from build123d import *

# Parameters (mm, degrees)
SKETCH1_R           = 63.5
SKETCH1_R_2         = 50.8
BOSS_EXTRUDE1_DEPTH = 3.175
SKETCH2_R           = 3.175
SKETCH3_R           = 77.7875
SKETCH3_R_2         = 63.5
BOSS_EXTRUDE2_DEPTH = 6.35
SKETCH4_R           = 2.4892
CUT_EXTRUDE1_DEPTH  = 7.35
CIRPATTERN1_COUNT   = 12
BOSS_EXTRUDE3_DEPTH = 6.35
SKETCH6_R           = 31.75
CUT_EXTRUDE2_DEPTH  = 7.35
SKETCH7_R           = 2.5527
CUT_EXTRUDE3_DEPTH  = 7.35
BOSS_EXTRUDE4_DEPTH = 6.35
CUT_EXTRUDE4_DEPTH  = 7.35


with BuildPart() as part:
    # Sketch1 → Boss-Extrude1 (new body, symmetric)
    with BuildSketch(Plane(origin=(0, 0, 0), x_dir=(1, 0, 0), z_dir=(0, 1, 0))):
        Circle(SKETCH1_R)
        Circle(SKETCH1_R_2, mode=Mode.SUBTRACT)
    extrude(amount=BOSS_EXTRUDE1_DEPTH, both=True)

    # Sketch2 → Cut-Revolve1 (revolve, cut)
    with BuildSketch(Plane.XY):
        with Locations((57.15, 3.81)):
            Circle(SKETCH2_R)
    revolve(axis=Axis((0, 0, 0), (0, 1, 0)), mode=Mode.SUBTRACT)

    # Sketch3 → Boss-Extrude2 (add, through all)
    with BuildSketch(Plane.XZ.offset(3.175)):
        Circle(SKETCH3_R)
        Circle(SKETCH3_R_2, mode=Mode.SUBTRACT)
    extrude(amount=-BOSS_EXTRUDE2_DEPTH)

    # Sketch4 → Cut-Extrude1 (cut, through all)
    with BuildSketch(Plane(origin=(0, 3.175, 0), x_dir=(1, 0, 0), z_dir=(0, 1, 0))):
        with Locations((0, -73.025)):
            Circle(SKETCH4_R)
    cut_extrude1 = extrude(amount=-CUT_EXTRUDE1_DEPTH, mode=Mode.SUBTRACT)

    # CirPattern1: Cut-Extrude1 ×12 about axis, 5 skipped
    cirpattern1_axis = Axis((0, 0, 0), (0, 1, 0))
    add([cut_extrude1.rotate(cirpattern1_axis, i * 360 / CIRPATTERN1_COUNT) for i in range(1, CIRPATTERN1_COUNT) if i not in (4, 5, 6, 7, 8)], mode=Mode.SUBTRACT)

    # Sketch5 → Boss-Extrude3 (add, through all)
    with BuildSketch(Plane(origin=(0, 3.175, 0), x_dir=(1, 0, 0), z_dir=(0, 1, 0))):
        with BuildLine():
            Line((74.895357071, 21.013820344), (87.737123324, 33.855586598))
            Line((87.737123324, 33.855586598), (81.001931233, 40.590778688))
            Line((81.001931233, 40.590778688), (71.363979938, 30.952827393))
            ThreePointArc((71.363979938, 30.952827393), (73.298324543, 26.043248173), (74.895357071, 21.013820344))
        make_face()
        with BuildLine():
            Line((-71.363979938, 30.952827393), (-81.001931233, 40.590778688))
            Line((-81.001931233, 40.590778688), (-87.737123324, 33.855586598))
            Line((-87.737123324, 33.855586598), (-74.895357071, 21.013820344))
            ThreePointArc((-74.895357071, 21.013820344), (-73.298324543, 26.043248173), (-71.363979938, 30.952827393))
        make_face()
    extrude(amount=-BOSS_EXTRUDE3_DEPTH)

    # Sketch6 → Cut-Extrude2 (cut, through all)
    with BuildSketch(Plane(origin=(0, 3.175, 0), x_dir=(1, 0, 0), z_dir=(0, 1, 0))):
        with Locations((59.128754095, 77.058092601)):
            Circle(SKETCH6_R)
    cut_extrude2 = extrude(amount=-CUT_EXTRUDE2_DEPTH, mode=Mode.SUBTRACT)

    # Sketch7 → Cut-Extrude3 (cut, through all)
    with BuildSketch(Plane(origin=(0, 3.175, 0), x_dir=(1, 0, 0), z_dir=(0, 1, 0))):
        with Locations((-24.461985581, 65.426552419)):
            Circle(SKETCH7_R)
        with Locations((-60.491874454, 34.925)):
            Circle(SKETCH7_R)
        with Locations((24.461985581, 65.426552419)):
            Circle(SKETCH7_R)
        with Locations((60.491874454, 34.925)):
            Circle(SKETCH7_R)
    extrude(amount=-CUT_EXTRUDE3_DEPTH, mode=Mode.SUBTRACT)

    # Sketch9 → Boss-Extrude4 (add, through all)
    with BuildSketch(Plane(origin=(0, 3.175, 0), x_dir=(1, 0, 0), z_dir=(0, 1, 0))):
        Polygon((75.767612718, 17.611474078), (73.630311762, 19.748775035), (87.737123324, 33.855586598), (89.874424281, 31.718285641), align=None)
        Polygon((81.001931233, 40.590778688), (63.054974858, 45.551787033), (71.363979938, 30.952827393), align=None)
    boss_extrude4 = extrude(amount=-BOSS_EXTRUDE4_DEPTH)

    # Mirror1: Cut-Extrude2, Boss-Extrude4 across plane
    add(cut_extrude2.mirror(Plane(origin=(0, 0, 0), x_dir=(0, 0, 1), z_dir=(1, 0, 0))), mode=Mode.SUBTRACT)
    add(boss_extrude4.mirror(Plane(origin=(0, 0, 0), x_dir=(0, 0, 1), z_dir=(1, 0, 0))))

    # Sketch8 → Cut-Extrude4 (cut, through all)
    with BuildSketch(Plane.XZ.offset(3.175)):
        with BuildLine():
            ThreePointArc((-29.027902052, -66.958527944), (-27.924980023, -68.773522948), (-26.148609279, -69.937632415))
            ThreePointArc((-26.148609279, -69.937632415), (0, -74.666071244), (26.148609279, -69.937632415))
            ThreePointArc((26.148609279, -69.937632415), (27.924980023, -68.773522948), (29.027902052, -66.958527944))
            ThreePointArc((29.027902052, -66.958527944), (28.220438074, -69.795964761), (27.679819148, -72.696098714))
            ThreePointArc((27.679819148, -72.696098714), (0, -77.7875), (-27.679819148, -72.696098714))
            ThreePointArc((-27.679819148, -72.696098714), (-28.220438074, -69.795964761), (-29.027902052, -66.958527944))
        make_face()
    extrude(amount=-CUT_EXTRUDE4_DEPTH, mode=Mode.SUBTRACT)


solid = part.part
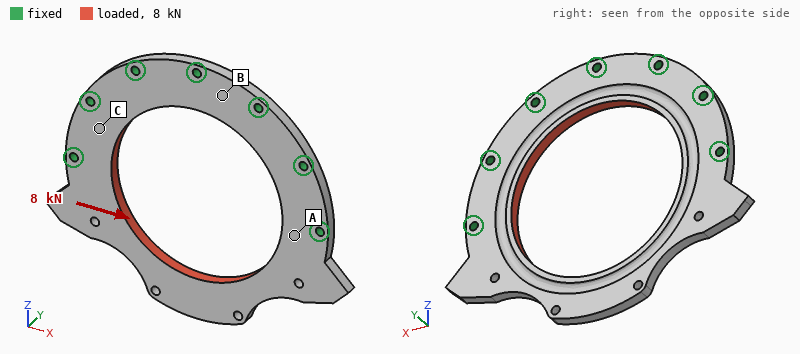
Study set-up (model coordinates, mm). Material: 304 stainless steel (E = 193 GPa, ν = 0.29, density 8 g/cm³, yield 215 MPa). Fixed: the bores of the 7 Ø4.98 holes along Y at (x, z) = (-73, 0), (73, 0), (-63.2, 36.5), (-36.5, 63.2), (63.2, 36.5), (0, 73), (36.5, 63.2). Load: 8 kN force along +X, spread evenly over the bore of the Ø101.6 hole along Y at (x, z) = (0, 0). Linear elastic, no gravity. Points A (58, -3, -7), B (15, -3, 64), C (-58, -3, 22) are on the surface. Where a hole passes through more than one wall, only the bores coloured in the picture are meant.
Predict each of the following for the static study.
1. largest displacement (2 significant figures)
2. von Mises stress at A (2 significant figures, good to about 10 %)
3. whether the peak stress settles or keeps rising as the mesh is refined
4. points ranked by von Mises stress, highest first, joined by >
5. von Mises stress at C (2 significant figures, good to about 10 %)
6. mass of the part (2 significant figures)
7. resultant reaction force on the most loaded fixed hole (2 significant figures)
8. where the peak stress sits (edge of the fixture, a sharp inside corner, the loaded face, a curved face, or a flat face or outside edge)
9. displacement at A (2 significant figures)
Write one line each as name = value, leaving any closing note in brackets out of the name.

largest displacement = 32 µm
von Mises stress at A = 27 MPa
whether the peak stress settles or keeps rising as the mesh is refined = keeps rising
points ranked by von Mises stress, highest first, joined by > = A > C > B
von Mises stress at C = 14 MPa
mass of the part = 490 g
resultant reaction force on the most loaded fixed hole = 3.2 kN
where the peak stress sits = edge of the fixture
displacement at A = 5.6 µm
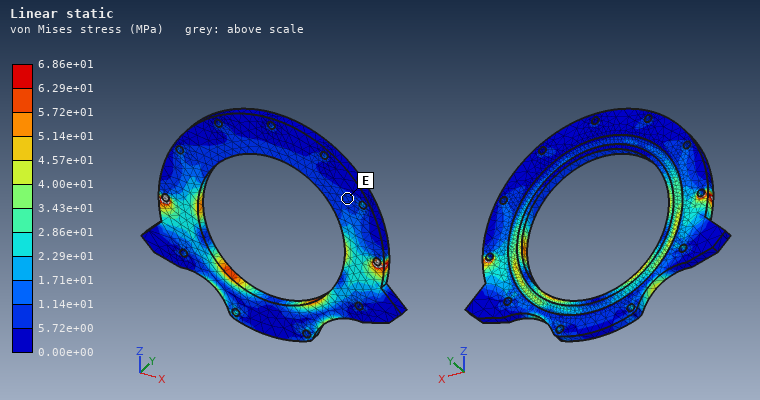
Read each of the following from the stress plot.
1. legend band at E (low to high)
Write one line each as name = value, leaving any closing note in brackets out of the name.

legend band at E = 5.72e+00 to 1.14e+01 MPa
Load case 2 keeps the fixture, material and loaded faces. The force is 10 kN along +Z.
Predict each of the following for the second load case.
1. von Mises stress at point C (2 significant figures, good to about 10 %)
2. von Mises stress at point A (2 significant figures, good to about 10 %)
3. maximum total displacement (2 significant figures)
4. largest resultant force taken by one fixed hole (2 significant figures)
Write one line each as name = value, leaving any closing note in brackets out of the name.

von Mises stress at point C = 14 MPa
von Mises stress at point A = 21 MPa
maximum total displacement = 20 µm
largest resultant force taken by one fixed hole = 2.3 kN
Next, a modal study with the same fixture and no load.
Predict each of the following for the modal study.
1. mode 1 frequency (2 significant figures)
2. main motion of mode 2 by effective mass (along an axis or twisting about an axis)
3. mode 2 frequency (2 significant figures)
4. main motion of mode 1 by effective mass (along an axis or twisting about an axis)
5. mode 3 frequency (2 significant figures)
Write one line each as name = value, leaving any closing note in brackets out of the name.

mode 1 frequency = 650 Hz
main motion of mode 2 by effective mass = twisting about Z
mode 2 frequency = 1800 Hz
main motion of mode 1 by effective mass = along Y
mode 3 frequency = 2800 Hz
